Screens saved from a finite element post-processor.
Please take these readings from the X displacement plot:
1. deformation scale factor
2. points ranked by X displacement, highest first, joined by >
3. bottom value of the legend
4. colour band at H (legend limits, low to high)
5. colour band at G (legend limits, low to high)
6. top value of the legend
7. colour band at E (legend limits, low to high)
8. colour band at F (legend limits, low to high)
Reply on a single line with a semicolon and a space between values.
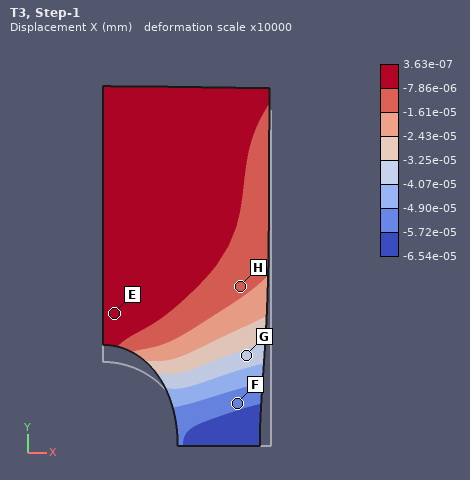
10000; E > H > G > F; -6.54e-05 mm; -1.61e-05 to -7.86e-06 mm; -4.07e-05 to -3.25e-05 mm; 3.63e-07 mm; -7.86e-06 to 3.63e-07 mm; -5.72e-05 to -4.90e-05 mm
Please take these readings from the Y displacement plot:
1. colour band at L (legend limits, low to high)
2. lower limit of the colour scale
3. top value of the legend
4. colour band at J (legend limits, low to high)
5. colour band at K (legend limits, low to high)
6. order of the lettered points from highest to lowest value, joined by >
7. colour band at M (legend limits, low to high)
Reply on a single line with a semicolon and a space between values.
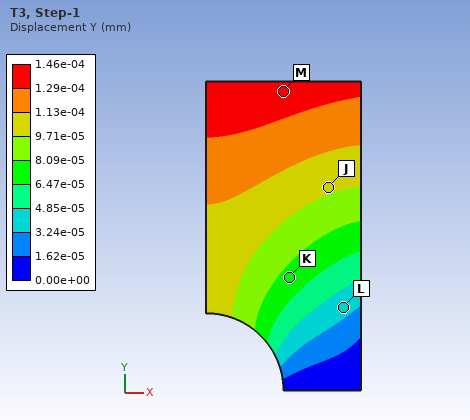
3.24e-05 to 4.85e-05 mm; 0.00e+00 mm; 1.46e-04 mm; 9.71e-05 to 1.13e-04 mm; 6.47e-05 to 8.09e-05 mm; M > J > K > L; 1.29e-04 to 1.46e-04 mm
